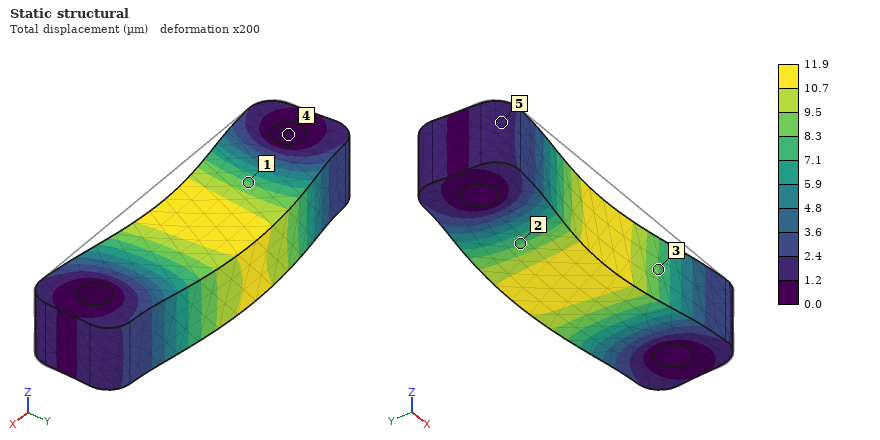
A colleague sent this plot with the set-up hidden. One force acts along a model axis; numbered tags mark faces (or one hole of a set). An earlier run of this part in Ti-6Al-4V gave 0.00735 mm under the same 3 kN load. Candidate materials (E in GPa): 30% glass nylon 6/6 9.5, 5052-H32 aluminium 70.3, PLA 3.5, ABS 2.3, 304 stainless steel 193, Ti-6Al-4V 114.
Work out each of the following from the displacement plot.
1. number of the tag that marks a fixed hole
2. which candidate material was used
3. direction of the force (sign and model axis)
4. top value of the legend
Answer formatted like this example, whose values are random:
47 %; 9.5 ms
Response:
4; 5052-H32 aluminium; +Y; 11.9 µm
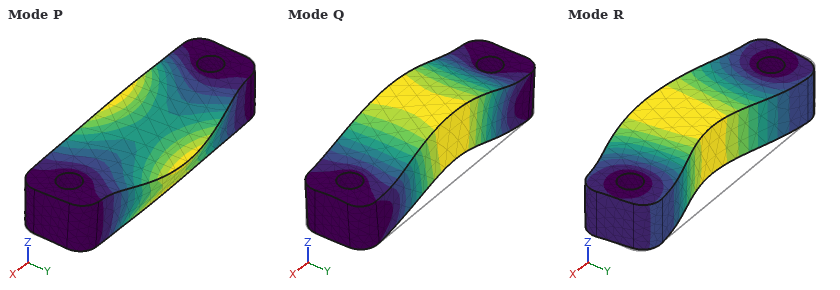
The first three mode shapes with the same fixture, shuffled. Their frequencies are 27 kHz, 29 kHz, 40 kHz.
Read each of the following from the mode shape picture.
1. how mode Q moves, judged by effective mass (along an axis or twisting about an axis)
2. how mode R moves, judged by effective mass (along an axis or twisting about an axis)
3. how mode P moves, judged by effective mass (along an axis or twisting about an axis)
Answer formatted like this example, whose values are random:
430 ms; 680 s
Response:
along Z; along Y; twisting about X
